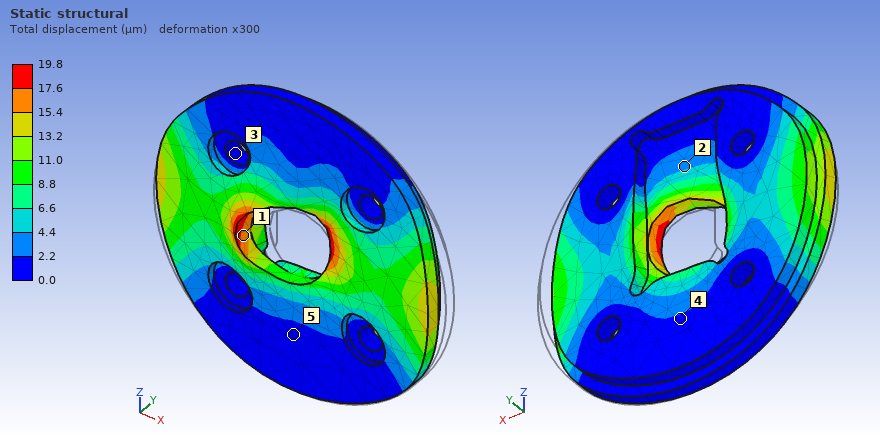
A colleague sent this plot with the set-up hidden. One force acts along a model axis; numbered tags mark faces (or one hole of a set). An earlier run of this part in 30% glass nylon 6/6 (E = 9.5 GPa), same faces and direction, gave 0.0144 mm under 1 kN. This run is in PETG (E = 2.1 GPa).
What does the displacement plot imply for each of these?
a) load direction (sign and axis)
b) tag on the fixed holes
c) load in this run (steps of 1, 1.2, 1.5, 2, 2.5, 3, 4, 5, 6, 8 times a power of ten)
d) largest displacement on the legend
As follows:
-X
3
300 N
19.8 µm
